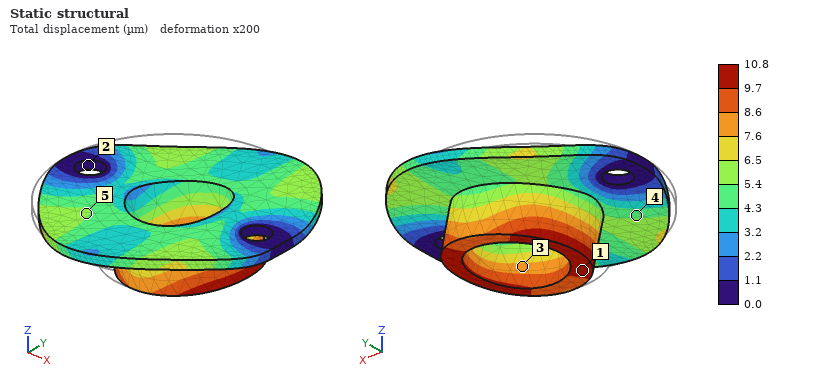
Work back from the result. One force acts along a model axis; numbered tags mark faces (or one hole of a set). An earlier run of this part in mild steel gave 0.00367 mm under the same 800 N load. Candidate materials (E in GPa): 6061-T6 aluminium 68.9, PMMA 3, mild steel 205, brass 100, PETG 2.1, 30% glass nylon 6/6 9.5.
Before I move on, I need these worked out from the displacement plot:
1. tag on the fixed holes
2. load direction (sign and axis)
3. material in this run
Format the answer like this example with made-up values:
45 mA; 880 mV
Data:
2; +X; 6061-T6 aluminium
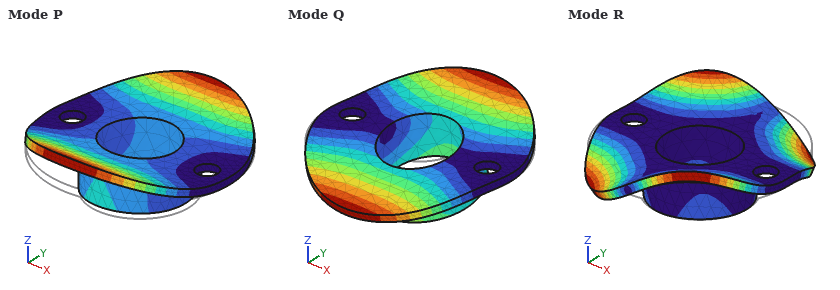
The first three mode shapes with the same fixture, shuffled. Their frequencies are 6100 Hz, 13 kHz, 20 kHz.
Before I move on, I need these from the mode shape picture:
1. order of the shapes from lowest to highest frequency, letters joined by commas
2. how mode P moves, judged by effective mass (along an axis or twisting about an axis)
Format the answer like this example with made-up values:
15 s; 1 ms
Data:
Q, P, R; along Z
